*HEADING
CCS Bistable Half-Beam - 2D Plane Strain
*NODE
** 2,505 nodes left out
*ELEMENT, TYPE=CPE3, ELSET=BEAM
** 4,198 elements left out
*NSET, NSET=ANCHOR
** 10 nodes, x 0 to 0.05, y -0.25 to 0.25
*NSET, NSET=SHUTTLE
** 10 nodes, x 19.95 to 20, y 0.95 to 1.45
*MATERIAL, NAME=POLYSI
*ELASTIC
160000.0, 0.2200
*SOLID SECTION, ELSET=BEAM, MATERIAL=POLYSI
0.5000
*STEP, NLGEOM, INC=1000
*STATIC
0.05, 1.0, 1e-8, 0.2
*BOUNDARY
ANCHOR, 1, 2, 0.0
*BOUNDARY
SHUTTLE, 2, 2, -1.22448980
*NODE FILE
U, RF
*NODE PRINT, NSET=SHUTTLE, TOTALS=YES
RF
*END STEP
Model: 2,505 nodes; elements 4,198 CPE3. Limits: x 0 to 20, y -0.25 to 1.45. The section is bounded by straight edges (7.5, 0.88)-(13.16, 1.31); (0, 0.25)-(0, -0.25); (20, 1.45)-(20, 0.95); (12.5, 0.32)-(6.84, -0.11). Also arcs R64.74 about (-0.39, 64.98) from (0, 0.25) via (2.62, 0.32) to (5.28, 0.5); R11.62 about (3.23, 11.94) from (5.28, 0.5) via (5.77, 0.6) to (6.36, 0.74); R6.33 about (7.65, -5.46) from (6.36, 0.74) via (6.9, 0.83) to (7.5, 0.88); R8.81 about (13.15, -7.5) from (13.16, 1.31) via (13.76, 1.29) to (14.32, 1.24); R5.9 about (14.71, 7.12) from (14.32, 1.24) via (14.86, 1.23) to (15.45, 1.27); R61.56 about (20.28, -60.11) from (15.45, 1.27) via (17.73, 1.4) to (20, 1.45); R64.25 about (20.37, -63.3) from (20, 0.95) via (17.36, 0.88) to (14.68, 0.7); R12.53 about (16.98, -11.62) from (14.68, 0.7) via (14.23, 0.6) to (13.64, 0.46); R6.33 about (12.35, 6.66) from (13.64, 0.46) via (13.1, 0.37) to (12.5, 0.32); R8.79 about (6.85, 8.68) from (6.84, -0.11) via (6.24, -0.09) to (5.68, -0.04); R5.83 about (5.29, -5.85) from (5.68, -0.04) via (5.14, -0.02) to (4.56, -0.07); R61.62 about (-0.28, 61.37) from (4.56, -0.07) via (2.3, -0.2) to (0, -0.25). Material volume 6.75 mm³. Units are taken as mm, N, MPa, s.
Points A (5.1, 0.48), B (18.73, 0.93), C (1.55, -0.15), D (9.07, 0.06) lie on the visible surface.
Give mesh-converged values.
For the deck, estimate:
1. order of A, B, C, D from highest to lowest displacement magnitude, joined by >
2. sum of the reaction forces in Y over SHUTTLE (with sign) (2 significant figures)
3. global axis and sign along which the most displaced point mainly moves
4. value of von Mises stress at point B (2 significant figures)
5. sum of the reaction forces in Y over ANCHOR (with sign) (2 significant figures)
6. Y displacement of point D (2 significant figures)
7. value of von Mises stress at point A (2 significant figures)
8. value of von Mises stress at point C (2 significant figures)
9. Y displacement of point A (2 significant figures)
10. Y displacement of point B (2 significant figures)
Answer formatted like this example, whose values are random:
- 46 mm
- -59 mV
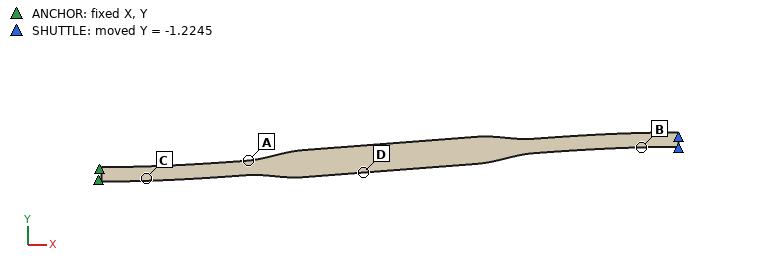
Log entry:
- B > D > A > C
- -1.1 N
- -Y
- 290 MPa
- 1.1 N
- -0.47 mm
- 380 MPa
- 370 MPa
- -0.18 mm
- -1.2 mm
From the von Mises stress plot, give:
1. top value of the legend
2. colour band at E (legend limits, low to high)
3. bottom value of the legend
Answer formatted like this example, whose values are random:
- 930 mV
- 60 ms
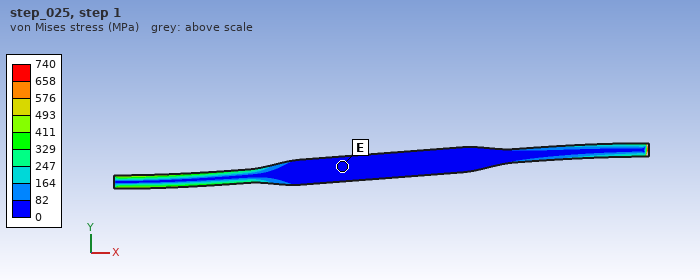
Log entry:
- 740 MPa
- 0 to 82 MPa
- 0 MPa
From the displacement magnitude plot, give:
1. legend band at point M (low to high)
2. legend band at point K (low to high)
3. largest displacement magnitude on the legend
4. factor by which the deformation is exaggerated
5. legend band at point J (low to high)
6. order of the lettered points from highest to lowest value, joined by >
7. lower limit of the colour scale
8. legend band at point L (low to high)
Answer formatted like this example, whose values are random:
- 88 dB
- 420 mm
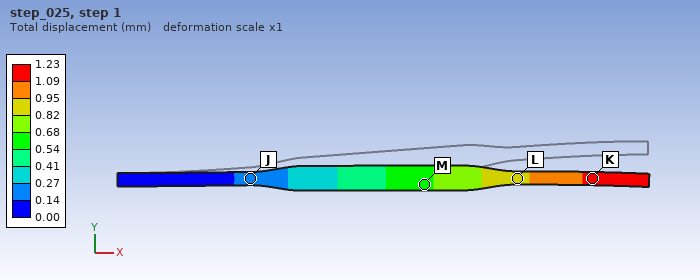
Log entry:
- 0.54 to 0.68 mm
- 1.09 to 1.23 mm
- 1.23 mm
- 1
- 0.14 to 0.27 mm
- K > L > M > J
- 0.00 mm
- 0.82 to 0.95 mm
